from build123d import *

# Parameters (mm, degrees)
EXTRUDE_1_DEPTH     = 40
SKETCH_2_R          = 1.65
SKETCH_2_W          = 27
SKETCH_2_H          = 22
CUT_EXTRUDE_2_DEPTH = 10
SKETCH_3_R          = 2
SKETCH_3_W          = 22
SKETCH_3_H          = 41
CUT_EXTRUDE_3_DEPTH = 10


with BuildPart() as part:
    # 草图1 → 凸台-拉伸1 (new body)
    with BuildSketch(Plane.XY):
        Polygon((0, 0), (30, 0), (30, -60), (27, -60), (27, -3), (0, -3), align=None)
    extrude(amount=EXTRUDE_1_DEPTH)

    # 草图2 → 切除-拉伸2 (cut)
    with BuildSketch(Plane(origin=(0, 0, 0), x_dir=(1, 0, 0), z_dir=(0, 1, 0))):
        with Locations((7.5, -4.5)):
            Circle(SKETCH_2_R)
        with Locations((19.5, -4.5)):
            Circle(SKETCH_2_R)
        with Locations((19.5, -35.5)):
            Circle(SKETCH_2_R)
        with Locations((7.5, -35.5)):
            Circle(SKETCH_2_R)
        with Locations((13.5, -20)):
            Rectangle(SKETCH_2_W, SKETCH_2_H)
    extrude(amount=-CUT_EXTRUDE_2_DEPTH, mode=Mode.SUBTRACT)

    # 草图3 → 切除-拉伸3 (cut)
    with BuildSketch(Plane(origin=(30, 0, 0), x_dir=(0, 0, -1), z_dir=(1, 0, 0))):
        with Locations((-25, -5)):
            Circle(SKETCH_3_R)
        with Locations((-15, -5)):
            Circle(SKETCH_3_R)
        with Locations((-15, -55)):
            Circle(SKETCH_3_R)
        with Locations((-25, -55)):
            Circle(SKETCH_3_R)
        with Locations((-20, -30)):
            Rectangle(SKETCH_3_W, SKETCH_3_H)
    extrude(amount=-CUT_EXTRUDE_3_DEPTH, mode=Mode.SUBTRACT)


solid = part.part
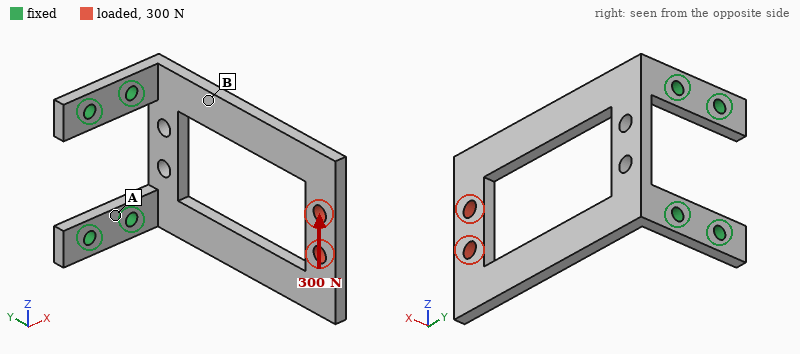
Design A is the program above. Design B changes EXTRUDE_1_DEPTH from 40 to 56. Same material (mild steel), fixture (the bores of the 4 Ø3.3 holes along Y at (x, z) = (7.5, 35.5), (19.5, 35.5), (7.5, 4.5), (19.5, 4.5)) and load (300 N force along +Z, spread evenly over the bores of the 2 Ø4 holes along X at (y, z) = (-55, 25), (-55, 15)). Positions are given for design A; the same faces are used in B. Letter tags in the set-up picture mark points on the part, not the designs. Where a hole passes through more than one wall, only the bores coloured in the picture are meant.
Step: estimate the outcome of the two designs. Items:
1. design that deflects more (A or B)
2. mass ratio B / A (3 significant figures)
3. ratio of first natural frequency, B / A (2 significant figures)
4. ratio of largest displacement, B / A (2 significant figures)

A
1.73
1.0
0.83
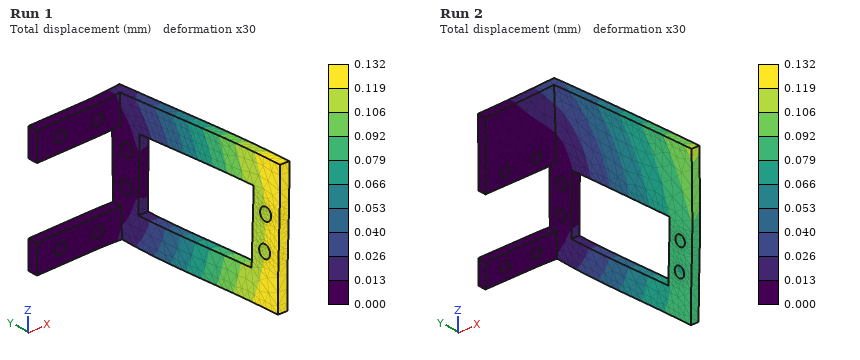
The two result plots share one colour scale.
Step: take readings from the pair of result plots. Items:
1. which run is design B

Run 2
